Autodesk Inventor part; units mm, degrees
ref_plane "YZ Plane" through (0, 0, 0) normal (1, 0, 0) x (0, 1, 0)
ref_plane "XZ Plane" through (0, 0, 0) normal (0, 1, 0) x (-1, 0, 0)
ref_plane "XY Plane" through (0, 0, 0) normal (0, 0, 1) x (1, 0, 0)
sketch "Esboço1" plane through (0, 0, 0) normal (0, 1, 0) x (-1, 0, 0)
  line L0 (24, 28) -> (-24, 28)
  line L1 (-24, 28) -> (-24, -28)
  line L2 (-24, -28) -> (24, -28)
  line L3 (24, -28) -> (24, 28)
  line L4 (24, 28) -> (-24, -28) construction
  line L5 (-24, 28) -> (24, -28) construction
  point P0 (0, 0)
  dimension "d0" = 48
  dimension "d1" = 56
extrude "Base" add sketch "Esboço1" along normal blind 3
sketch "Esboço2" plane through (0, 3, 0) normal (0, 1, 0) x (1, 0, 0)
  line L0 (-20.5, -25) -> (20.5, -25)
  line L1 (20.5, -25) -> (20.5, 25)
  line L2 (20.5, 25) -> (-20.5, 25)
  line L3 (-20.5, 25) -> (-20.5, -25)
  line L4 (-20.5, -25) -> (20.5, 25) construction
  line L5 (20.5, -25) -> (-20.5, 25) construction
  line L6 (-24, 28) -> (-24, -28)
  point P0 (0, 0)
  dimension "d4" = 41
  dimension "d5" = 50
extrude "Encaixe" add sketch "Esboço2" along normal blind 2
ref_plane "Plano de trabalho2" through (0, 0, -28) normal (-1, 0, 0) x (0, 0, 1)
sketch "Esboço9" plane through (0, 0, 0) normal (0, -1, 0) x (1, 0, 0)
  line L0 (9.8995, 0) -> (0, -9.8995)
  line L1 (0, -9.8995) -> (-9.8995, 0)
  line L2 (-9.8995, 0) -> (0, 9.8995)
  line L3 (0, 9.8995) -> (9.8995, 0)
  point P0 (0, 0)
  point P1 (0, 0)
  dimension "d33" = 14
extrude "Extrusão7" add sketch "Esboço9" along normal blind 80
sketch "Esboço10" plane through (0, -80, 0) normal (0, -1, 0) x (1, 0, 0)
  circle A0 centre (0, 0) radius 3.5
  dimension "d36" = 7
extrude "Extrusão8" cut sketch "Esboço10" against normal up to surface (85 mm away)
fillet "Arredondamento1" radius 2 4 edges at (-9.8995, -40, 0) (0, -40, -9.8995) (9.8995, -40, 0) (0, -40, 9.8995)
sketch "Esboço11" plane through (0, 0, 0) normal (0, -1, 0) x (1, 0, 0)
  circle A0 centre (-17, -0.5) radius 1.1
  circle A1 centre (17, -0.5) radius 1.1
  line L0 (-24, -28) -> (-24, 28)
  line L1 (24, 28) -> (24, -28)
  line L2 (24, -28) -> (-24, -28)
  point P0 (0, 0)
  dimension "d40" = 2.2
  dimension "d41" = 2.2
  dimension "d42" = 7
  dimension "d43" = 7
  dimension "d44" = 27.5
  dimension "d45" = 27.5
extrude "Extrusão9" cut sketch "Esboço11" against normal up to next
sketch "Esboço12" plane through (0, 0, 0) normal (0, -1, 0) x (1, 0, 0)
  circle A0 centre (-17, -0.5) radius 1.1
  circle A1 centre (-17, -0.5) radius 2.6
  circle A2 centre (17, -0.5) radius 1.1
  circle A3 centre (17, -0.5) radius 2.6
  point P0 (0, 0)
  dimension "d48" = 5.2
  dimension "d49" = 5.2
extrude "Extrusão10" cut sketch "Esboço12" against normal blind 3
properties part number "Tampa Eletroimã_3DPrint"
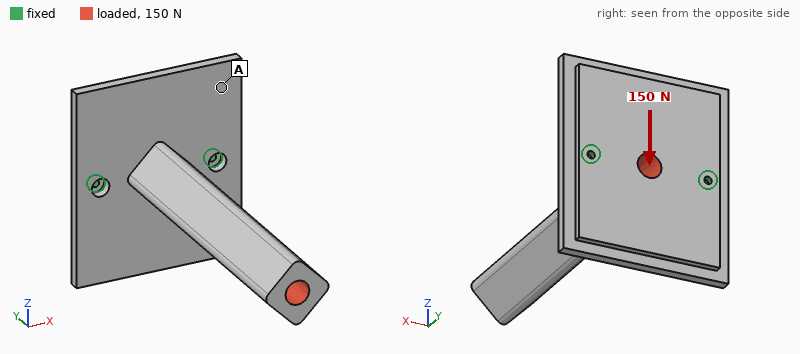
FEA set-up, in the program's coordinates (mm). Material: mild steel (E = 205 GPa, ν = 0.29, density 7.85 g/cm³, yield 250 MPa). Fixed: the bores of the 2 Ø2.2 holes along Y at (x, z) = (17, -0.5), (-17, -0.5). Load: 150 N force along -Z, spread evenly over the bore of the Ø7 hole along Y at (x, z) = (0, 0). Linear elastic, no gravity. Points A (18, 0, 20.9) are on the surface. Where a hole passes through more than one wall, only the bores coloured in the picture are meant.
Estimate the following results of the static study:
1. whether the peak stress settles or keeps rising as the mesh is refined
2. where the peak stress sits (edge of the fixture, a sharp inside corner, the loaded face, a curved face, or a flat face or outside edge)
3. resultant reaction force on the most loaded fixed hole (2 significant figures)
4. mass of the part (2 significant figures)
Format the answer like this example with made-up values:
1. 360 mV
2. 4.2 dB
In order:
1. keeps rising
2. edge of the fixture
3. 75 N
4. 190 g
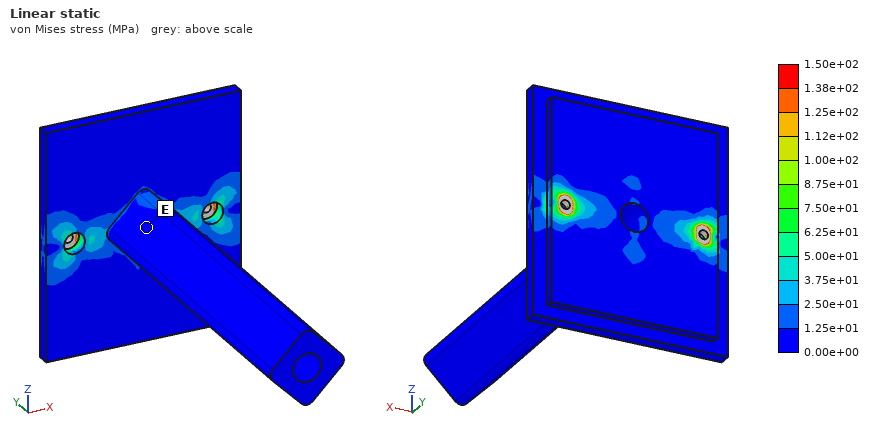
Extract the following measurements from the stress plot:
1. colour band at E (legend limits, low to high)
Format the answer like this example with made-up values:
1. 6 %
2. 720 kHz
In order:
1. 0.00e+00 to 1.25e+01 MPa
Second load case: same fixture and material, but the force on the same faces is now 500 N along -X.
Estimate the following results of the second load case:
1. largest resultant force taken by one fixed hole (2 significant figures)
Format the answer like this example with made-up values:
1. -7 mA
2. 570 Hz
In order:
1. 690 N
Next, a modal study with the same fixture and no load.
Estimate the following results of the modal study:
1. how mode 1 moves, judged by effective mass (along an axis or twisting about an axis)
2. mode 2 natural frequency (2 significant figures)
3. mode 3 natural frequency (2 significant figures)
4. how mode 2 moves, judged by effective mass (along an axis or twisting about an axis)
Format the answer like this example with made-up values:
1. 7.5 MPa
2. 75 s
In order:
1. along Z
2. 1400 Hz
3. 4400 Hz
4. along X
